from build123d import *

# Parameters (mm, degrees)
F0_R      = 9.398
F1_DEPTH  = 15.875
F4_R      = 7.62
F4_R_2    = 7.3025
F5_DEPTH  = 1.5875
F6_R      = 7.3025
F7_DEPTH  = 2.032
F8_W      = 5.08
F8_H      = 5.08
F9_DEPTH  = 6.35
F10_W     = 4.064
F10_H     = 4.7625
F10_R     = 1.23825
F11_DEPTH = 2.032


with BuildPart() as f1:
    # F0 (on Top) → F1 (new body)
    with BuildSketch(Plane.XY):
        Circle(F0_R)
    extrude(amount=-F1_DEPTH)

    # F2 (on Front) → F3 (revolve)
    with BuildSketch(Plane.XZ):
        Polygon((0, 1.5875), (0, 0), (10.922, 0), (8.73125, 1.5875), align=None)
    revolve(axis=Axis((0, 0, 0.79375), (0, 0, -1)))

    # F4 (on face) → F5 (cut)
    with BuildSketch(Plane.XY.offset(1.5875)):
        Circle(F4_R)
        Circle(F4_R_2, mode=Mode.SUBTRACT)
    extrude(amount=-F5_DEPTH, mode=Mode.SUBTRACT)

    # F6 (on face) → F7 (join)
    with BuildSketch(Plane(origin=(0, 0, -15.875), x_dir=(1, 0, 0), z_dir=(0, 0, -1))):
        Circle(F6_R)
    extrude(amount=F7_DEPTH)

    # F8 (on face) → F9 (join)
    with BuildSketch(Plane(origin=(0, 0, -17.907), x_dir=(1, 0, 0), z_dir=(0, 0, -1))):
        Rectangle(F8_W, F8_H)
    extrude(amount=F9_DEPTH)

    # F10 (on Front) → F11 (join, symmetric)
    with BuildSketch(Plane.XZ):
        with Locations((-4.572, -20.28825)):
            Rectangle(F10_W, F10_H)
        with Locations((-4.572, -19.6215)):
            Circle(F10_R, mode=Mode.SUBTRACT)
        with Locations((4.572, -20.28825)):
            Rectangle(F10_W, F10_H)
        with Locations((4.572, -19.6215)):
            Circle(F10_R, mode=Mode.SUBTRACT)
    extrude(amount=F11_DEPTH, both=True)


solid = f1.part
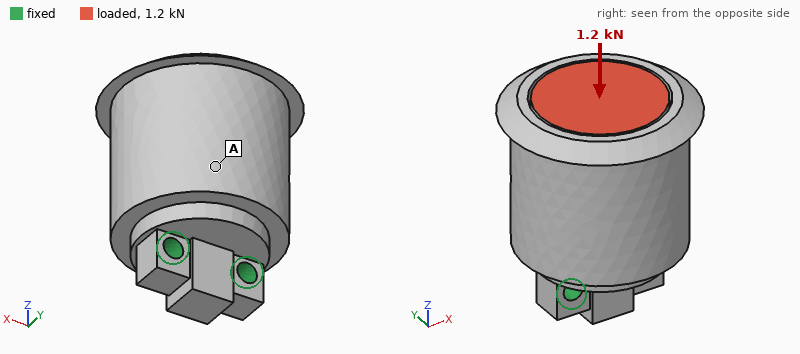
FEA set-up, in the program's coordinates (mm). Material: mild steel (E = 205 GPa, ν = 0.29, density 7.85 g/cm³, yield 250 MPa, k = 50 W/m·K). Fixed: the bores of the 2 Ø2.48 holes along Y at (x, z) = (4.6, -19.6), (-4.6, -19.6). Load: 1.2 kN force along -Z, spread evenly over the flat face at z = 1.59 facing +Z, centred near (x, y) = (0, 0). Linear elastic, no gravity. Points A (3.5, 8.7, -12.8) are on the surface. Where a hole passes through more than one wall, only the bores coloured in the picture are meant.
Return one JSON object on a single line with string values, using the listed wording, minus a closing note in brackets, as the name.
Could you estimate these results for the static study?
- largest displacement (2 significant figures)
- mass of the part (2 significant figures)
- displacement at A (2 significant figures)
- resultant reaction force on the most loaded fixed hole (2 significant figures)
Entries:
{"largest displacement": "0.95 µm", "mass of the part": "43 g", "displacement at A": "0.62 µm", "resultant reaction force on the most loaded fixed hole": "600 N"}
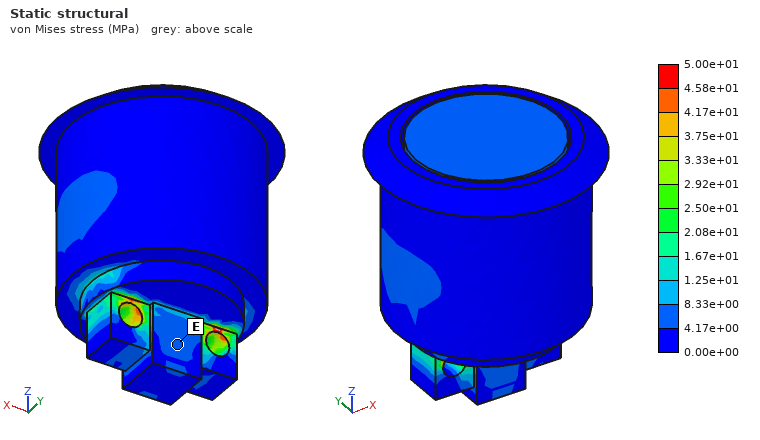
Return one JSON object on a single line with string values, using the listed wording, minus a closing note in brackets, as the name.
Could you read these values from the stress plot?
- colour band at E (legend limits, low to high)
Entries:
{"colour band at E": "4.17e+00 to 8.33e+00 MPa"}
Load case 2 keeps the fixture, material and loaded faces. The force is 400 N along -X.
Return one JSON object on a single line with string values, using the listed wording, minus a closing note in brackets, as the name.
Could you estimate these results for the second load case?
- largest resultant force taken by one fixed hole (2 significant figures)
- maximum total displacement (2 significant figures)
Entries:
{"largest resultant force taken by one fixed hole": "860 N", "maximum total displacement": "4.6 µm"}
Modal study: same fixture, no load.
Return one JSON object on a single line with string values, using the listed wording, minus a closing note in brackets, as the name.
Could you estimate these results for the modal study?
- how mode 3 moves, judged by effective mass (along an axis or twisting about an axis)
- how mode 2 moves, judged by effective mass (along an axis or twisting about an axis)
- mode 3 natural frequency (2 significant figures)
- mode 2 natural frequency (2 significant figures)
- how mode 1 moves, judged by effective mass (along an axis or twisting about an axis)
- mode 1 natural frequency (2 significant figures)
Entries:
{"how mode 3 moves, judged by effective mass": "twisting about Z", "how mode 2 moves, judged by effective mass": "along X", "mode 3 natural frequency": "18 kHz", "mode 2 natural frequency": "12 kHz", "how mode 1 moves, judged by effective mass": "along Y", "mode 1 natural frequency": "4800 Hz"}
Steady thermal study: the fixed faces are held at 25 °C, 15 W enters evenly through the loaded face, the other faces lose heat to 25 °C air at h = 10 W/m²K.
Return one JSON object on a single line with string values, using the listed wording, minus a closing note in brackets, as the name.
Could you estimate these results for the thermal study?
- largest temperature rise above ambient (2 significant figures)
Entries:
{"largest temperature rise above ambient": "38 K"}
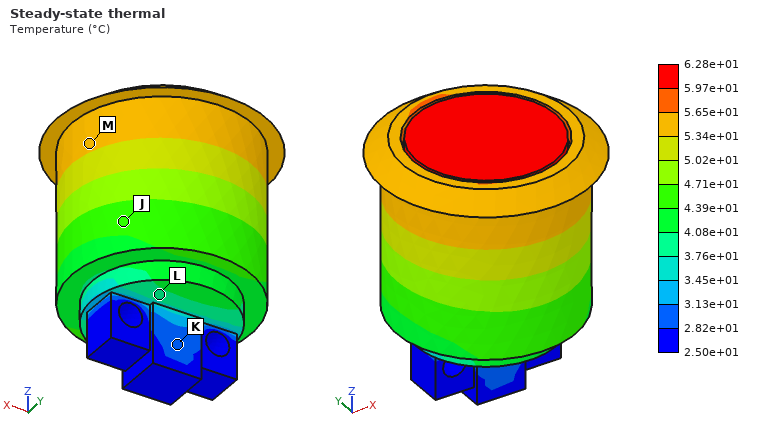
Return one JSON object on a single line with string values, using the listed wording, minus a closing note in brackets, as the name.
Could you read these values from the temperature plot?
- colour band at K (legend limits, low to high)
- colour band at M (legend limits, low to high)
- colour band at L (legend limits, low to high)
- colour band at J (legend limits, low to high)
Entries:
{"colour band at K": "2.82e+01 to 3.13e+01 °C", "colour band at M": "5.34e+01 to 5.65e+01 °C", "colour band at L": "3.76e+01 to 4.08e+01 °C", "colour band at J": "4.39e+01 to 4.71e+01 °C"}
